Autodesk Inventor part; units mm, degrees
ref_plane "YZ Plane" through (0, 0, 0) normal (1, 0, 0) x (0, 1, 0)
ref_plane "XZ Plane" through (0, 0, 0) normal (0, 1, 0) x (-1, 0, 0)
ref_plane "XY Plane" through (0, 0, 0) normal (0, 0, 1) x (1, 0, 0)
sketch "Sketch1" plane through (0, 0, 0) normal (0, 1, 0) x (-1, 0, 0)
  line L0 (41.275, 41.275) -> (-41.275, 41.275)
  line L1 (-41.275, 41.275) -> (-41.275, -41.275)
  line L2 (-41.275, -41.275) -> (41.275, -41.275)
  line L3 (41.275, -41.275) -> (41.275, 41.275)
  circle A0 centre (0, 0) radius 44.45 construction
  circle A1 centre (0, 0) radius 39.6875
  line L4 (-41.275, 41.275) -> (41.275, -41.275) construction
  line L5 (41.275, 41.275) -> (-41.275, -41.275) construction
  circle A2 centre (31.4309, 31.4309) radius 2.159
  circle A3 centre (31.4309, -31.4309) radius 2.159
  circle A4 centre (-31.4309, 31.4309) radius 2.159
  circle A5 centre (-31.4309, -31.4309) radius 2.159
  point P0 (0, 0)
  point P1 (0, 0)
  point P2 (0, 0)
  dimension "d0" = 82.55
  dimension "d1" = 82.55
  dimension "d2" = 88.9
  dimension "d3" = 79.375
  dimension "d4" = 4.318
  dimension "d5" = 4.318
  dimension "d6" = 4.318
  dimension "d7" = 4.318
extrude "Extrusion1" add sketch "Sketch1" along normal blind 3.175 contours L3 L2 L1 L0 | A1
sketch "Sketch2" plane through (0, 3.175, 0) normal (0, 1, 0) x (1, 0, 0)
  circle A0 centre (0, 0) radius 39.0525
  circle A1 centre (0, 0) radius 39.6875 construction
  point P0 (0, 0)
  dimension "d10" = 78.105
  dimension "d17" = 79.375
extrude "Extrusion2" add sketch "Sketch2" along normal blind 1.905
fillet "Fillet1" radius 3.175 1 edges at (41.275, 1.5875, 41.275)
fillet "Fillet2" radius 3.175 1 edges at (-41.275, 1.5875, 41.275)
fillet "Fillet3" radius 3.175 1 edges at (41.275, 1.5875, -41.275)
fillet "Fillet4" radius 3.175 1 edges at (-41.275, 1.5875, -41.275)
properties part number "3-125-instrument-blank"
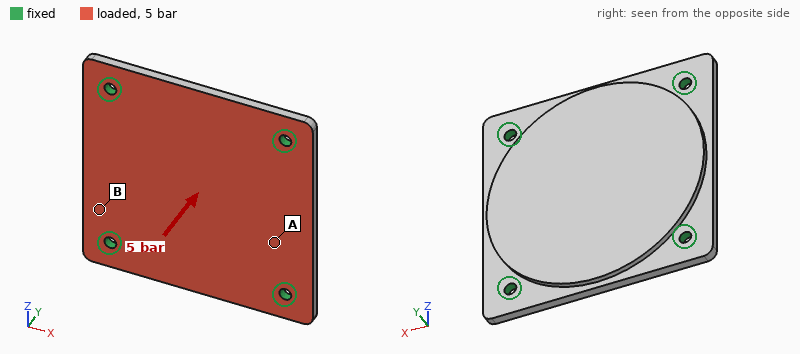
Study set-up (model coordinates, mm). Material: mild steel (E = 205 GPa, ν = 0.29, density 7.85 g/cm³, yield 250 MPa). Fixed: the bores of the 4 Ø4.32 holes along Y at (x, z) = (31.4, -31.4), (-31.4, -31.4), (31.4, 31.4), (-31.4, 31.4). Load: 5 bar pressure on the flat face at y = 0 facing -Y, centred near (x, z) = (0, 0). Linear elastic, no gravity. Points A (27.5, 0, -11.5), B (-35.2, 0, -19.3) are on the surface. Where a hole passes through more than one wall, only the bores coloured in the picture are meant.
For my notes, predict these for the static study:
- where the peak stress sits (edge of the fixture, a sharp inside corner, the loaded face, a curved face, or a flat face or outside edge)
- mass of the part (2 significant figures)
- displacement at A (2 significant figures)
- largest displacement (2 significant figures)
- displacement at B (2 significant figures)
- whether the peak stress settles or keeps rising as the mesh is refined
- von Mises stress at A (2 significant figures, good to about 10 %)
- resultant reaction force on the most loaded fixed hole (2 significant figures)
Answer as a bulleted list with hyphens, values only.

- edge of the fixture
- 240 g
- 20 µm
- 35 µm
- 9.2 µm
- keeps rising
- 22 MPa
- 1.2 kN
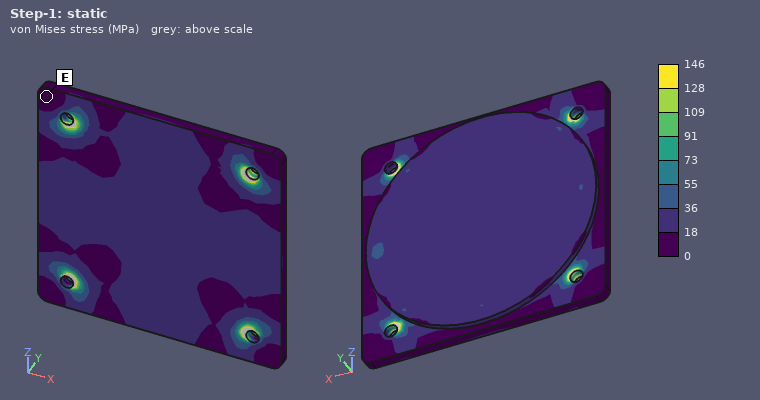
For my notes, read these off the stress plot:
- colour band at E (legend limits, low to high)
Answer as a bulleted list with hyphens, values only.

- 0 to 18 MPa
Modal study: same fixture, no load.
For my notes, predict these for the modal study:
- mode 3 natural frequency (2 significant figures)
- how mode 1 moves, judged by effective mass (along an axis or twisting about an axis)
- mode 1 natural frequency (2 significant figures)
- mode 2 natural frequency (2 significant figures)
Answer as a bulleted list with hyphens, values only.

- 5700 Hz
- along Y
- 3600 Hz
- 5700 Hz
